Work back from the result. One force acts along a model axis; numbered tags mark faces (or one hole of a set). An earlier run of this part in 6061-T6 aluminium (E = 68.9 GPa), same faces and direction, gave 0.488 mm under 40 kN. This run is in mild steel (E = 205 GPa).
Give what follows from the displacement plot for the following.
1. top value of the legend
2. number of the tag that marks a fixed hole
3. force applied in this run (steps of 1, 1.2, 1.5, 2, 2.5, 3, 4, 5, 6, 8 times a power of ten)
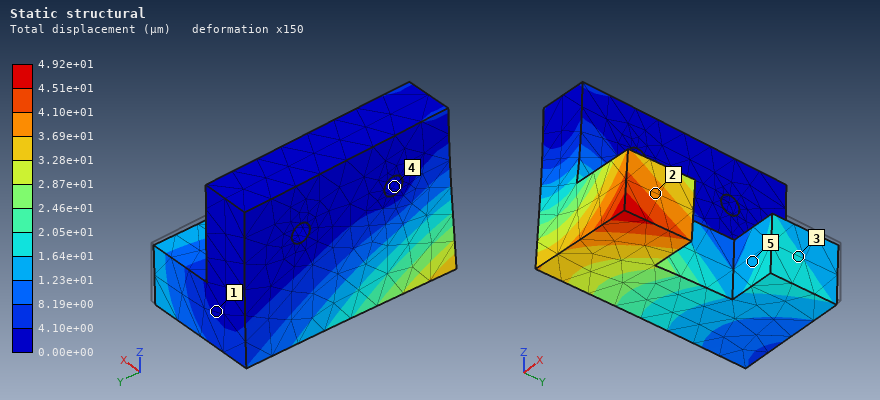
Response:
4.92e+01 µm
4
12 kN
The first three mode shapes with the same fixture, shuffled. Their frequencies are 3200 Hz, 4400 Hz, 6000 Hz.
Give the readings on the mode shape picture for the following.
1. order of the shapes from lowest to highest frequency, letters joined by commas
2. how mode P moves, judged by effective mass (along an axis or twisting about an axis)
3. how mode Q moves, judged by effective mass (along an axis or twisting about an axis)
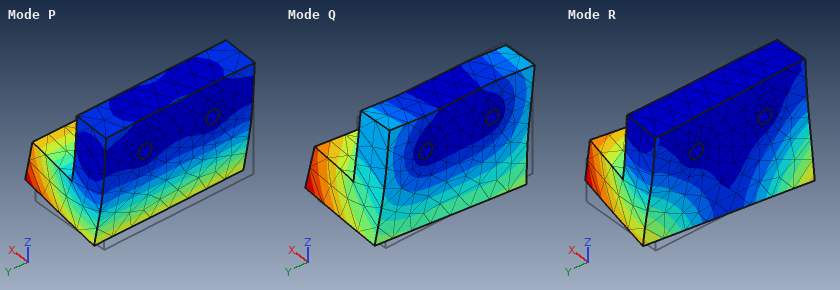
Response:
P, R, Q
along X
along Y
